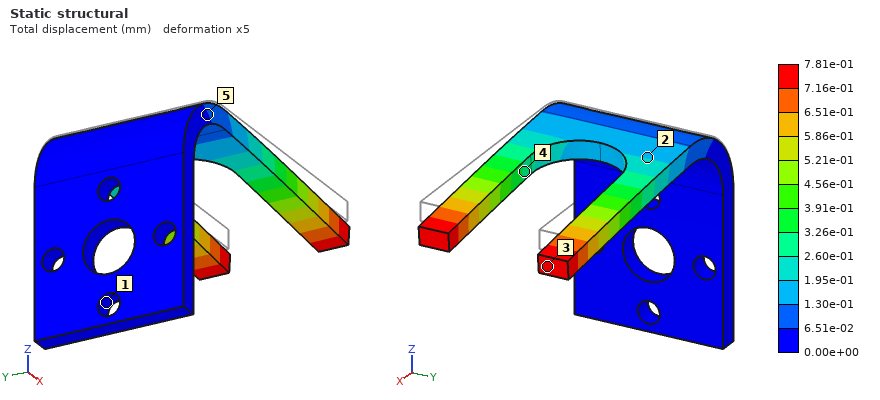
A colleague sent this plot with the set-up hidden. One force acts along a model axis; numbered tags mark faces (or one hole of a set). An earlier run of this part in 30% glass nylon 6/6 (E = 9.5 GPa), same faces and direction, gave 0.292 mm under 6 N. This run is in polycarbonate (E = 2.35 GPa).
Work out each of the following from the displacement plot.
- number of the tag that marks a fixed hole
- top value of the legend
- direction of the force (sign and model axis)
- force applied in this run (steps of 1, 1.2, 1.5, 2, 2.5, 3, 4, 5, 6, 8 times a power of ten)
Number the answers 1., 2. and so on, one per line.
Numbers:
1. 1
2. 7.81e-01 mm
3. -Z
4. 4 N
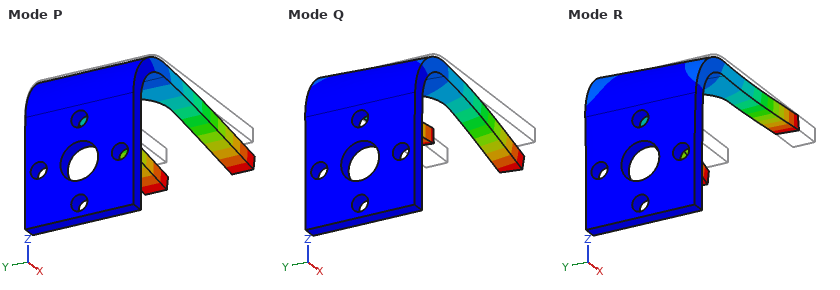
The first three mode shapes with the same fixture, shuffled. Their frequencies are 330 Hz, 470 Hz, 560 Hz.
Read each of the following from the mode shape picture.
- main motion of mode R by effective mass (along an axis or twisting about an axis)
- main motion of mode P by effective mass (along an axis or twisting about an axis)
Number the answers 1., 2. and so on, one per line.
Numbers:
1. along Y
2. along Z
